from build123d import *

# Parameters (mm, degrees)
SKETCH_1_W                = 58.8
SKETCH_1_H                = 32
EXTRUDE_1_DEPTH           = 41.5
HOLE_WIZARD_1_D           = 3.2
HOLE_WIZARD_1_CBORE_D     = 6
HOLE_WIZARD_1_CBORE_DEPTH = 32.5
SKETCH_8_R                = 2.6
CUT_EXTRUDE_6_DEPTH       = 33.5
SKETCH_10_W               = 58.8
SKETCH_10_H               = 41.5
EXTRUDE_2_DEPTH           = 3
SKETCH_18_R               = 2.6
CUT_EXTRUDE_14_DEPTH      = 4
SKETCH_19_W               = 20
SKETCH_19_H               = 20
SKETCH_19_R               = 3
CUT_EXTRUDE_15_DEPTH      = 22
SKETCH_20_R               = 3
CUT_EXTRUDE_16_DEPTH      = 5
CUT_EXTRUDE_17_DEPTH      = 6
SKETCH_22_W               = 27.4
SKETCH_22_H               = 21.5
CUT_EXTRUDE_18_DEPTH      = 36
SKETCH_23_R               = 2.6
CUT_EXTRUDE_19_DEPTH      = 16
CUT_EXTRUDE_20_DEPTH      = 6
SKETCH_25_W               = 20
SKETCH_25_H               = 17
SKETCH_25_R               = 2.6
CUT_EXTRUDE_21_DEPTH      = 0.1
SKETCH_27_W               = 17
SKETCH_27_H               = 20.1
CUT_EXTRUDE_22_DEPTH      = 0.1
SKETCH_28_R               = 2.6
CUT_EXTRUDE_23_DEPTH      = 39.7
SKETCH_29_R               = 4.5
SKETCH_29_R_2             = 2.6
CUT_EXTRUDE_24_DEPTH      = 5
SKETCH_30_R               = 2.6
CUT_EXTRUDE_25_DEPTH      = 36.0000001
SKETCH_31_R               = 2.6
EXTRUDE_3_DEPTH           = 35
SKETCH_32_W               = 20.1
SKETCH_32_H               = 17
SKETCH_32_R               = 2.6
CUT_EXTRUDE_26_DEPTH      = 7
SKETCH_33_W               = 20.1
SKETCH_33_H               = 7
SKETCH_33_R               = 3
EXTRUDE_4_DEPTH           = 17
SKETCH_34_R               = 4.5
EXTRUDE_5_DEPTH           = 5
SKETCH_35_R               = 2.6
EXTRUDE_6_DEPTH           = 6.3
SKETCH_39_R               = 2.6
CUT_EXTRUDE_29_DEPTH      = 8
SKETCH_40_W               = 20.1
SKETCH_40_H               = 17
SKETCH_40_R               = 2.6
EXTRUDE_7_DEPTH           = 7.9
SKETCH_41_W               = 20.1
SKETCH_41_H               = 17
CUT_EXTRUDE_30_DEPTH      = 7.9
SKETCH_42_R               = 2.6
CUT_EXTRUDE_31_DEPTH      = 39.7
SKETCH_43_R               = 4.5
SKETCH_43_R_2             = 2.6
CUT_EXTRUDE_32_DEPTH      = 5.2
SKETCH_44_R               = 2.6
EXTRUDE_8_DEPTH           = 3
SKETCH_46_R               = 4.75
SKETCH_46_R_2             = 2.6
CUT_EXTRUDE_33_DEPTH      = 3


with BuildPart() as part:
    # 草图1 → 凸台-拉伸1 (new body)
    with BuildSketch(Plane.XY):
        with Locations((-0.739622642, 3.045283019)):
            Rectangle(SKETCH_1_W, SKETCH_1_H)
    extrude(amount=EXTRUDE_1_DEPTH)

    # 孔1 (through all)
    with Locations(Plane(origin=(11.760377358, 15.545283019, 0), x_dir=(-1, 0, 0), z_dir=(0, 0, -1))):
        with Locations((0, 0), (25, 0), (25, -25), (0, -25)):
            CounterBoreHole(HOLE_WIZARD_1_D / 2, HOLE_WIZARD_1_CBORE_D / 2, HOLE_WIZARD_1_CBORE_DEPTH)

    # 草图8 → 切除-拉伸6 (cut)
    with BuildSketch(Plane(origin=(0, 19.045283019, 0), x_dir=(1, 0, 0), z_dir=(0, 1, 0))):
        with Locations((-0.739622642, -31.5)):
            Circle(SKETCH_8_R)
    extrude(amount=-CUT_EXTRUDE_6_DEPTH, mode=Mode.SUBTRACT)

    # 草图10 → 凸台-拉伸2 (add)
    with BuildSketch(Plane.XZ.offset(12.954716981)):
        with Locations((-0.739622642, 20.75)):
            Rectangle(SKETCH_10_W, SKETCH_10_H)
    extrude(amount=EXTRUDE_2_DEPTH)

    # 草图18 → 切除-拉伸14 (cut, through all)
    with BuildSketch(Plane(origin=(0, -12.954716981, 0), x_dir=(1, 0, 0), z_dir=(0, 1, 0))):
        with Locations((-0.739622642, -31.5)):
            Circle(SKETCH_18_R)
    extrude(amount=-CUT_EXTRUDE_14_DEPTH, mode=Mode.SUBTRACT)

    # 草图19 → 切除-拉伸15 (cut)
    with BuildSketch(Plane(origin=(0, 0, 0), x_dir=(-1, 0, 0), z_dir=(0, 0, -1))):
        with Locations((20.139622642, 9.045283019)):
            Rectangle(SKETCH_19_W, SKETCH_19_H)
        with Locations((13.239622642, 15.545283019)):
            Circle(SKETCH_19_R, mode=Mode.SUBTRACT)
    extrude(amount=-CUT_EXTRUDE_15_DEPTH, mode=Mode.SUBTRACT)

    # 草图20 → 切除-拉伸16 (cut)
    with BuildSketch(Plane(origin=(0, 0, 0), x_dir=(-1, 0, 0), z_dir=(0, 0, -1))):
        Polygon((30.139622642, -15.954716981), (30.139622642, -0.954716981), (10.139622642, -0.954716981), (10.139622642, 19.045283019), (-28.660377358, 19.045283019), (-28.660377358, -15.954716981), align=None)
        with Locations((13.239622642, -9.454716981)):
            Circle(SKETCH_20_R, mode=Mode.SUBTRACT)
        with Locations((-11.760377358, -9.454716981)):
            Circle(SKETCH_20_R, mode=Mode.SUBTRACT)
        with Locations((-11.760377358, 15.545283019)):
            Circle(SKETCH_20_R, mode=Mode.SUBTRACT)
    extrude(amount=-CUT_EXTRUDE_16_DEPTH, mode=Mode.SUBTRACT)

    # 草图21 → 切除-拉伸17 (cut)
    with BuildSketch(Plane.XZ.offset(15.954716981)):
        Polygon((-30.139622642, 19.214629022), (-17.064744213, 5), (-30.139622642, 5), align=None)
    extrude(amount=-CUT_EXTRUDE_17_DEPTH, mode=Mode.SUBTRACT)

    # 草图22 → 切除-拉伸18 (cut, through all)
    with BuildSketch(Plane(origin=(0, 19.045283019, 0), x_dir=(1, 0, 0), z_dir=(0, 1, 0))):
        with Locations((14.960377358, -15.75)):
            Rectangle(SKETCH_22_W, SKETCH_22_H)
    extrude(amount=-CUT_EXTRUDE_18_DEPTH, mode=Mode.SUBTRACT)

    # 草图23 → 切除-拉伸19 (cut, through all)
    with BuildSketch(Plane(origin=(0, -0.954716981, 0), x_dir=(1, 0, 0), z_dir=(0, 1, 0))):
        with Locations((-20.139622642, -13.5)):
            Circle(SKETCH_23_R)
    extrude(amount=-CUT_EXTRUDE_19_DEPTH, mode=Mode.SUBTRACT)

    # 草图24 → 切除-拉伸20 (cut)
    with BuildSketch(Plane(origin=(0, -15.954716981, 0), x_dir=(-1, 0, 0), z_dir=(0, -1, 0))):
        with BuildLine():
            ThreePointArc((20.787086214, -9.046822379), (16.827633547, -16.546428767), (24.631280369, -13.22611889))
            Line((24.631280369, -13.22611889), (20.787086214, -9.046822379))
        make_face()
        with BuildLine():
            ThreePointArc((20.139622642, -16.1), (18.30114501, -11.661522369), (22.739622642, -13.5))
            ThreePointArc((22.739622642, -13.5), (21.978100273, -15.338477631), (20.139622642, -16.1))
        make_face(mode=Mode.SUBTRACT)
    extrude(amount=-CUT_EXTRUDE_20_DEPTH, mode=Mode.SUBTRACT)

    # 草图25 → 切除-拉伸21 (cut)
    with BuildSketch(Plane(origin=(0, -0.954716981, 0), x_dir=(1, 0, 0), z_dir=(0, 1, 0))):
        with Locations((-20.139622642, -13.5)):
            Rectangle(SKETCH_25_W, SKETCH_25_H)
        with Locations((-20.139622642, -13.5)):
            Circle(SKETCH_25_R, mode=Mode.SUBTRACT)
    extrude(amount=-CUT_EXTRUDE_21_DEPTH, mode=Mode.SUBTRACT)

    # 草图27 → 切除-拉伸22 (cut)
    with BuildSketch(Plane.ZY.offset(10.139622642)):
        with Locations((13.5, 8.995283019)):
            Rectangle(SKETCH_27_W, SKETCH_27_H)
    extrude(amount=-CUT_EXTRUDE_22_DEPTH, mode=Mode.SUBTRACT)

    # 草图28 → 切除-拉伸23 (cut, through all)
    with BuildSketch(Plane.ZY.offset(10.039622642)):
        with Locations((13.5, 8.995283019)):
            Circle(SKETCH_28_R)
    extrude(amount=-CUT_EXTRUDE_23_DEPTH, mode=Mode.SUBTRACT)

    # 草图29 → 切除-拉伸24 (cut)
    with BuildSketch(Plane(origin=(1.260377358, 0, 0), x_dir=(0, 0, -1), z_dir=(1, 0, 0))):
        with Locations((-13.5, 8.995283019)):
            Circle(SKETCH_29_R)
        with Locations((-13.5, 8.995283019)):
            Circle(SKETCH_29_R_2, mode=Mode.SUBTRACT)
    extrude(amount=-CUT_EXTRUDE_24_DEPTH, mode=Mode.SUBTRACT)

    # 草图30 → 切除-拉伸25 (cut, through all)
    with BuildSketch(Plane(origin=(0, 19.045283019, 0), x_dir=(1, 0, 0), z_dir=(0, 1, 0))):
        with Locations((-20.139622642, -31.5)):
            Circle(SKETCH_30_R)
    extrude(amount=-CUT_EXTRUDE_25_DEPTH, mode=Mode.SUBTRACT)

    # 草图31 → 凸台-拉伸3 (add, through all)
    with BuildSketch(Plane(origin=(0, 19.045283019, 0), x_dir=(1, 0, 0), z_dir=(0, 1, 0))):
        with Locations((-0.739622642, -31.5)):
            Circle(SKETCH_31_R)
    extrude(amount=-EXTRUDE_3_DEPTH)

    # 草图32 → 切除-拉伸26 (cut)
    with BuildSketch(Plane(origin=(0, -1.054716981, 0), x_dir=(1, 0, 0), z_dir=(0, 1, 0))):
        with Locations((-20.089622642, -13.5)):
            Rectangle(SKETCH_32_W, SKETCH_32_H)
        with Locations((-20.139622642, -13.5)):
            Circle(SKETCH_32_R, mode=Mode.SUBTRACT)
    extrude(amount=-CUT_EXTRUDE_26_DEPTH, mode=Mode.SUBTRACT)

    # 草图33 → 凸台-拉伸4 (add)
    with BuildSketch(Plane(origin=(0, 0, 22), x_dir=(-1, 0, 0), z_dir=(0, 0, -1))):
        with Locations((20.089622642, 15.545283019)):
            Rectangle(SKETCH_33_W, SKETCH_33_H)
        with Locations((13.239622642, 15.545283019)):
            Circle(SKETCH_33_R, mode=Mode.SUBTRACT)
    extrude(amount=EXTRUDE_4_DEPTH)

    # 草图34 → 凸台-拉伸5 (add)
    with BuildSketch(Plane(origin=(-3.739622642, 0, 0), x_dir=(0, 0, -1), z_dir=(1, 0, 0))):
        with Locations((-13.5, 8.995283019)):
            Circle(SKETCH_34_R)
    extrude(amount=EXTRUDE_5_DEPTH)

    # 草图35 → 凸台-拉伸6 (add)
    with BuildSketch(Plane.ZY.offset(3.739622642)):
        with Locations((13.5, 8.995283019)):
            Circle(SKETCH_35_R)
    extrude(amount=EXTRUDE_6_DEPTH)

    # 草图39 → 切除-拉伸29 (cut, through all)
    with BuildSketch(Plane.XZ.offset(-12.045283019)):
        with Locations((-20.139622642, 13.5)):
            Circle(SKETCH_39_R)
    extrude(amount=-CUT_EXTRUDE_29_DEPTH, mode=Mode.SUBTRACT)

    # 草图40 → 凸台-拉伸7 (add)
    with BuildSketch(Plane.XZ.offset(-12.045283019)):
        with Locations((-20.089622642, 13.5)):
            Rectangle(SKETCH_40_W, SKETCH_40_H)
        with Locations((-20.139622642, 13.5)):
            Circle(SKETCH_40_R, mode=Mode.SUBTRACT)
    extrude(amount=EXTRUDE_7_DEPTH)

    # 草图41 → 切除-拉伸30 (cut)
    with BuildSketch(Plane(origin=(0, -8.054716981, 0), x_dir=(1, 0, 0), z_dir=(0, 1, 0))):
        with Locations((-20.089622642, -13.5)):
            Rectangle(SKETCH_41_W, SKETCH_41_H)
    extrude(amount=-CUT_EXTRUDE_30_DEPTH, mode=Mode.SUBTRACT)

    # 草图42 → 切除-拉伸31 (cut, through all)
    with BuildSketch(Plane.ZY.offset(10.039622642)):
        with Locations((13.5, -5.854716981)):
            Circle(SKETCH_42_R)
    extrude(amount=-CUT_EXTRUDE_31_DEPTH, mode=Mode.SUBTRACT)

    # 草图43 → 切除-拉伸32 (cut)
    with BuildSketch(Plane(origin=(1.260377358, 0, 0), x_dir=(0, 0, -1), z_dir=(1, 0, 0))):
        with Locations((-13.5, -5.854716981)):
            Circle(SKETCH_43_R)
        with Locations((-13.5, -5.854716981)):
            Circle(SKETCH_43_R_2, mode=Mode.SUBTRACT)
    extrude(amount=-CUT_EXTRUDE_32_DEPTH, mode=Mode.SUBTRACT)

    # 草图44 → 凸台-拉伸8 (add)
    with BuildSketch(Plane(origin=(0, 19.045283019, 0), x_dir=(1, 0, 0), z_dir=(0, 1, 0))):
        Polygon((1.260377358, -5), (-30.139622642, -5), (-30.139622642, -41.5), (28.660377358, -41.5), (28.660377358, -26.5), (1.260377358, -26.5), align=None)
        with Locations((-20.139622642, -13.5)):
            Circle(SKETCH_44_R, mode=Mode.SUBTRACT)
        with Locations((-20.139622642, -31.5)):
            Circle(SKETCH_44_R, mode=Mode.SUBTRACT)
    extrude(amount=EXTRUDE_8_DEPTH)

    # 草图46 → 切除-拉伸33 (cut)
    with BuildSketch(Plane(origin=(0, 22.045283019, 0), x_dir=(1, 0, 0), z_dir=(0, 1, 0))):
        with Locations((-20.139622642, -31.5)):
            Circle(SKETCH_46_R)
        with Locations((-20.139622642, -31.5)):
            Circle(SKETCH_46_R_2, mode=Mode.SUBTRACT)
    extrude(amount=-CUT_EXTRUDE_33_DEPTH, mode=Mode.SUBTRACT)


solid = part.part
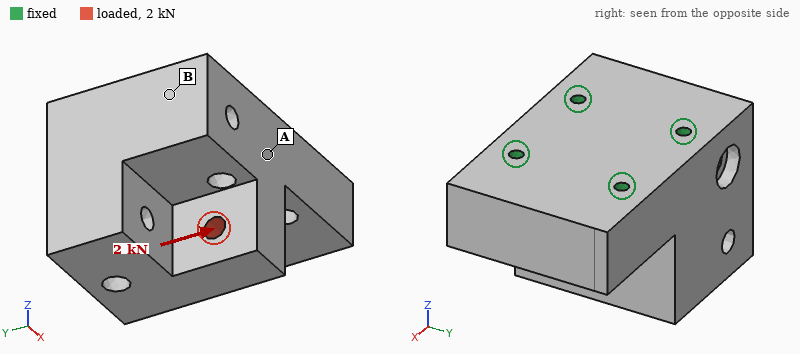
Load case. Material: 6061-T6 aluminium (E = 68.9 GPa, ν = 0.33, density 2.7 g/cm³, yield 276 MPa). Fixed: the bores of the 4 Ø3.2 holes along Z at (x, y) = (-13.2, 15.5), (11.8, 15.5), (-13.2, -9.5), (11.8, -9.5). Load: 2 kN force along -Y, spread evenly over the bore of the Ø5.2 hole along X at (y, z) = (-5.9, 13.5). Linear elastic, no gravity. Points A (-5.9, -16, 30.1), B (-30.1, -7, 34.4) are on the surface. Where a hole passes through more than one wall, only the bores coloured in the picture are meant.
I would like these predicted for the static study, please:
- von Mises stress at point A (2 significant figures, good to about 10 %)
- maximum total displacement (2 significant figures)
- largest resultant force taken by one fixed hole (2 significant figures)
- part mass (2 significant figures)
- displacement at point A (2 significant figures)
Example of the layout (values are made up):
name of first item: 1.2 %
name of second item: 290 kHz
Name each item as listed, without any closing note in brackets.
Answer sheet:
von Mises stress at point A: 8.2 MPa
maximum total displacement: 12 µm
largest resultant force taken by one fixed hole: 1.3 kN
part mass: 130 g
displacement at point A: 3.6 µm
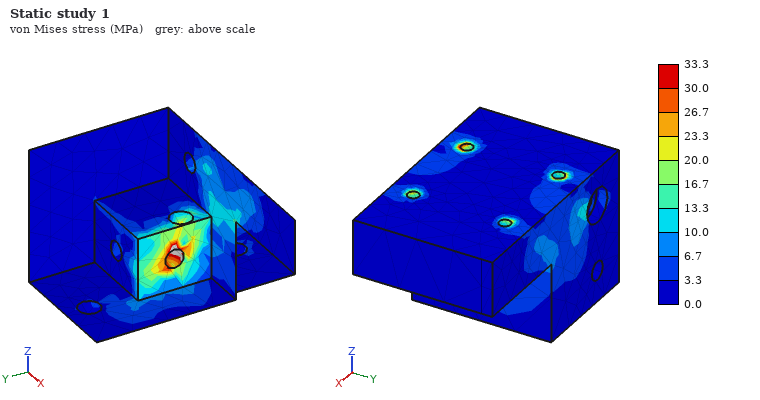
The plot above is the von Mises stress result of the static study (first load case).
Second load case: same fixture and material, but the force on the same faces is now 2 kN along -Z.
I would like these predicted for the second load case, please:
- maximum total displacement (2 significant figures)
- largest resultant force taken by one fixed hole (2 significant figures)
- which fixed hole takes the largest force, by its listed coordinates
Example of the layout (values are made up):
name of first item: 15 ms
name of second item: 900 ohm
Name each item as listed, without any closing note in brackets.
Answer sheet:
maximum total displacement: 6.9 µm
largest resultant force taken by one fixed hole: 1.2 kN
which fixed hole takes the largest force, by its listed coordinates: (-13.2, -9.5)
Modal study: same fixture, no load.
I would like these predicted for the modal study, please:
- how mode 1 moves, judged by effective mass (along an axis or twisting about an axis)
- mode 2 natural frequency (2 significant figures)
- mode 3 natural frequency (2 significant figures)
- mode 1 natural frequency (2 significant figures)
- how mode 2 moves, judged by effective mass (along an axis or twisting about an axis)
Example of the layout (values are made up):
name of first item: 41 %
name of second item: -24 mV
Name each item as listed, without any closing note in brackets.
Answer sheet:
how mode 1 moves, judged by effective mass: along X
mode 2 natural frequency: 13 kHz
mode 3 natural frequency: 19 kHz
mode 1 natural frequency: 11 kHz
how mode 2 moves, judged by effective mass: along Y
